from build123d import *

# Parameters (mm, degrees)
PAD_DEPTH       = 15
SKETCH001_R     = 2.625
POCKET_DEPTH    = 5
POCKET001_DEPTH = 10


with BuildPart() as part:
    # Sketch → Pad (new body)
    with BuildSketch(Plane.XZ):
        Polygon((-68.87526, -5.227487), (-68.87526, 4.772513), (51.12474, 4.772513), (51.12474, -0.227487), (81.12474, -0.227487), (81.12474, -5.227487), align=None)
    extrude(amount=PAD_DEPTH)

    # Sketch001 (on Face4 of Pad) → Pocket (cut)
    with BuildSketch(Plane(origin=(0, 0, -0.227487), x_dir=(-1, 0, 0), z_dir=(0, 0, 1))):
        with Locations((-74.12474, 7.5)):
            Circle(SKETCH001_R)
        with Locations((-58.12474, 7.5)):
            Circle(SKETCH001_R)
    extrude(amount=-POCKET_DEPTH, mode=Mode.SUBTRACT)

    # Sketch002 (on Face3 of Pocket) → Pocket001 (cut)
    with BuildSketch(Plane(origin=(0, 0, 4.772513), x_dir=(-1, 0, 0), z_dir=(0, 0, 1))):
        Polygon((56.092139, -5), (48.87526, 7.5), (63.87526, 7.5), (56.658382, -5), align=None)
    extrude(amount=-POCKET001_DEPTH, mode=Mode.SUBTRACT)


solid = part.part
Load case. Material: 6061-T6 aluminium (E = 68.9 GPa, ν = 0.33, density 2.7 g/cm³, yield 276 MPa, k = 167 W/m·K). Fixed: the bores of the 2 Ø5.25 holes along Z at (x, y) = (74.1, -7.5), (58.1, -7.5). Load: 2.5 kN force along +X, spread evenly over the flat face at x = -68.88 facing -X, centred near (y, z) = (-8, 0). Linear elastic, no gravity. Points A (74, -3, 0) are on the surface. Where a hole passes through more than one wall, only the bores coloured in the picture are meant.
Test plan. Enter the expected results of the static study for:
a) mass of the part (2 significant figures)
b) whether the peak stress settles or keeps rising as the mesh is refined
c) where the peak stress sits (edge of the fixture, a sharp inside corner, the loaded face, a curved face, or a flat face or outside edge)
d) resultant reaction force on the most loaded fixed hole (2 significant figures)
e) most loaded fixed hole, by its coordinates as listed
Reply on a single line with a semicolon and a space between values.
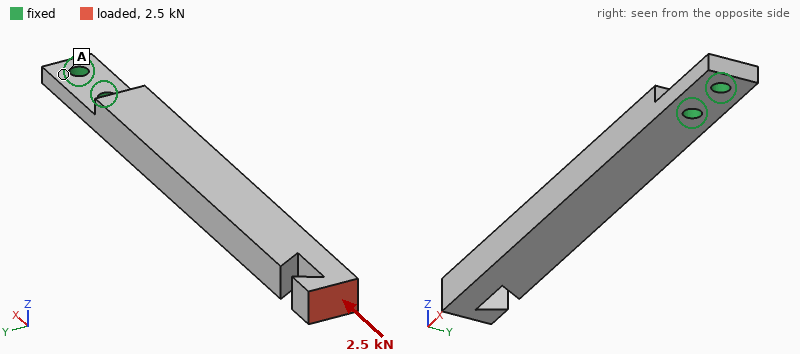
52 g; keeps rising; edge of the fixture; 2.3 kN; (58.1, -7.5)
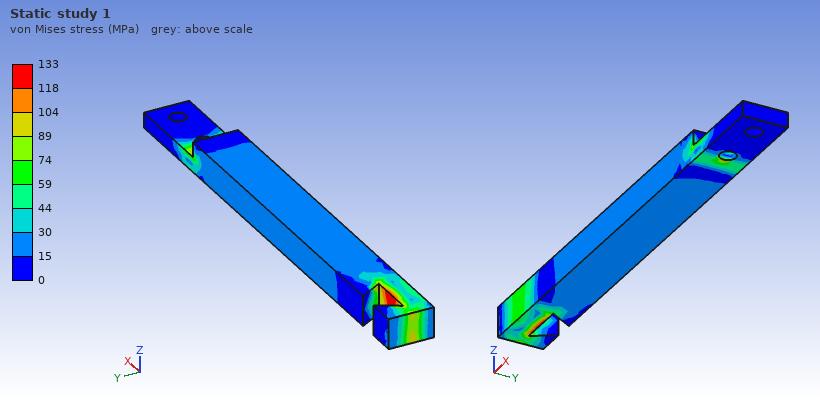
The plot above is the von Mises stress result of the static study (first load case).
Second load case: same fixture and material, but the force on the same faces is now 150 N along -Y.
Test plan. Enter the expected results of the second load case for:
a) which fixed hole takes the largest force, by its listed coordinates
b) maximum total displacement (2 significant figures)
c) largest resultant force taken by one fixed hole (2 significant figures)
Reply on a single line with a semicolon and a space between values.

(58.1, -7.5); 0.78 mm; 650 N
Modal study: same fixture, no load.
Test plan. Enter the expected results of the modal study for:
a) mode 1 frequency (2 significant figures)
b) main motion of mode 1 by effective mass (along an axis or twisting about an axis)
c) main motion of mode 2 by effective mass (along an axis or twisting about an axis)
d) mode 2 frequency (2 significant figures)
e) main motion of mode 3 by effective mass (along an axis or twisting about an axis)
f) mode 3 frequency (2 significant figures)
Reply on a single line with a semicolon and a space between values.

340 Hz; along Z; along Y; 640 Hz; along Z; 2600 Hz
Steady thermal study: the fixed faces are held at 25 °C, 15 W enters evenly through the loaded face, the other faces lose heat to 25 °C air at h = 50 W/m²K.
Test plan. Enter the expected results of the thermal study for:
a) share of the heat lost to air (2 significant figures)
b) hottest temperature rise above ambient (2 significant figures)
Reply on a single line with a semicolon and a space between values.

53 %; 64 K
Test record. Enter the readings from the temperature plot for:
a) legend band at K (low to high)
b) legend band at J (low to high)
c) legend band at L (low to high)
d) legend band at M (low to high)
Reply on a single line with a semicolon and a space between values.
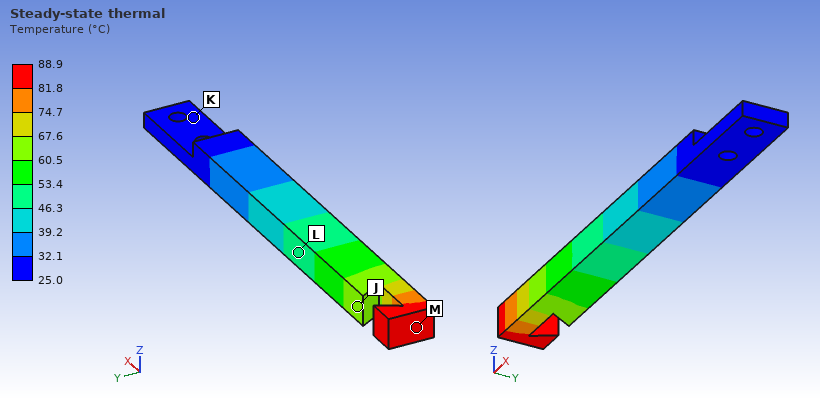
25.0 to 32.1 °C; 60.5 to 67.6 °C; 46.3 to 53.4 °C; 81.8 to 88.9 °C
